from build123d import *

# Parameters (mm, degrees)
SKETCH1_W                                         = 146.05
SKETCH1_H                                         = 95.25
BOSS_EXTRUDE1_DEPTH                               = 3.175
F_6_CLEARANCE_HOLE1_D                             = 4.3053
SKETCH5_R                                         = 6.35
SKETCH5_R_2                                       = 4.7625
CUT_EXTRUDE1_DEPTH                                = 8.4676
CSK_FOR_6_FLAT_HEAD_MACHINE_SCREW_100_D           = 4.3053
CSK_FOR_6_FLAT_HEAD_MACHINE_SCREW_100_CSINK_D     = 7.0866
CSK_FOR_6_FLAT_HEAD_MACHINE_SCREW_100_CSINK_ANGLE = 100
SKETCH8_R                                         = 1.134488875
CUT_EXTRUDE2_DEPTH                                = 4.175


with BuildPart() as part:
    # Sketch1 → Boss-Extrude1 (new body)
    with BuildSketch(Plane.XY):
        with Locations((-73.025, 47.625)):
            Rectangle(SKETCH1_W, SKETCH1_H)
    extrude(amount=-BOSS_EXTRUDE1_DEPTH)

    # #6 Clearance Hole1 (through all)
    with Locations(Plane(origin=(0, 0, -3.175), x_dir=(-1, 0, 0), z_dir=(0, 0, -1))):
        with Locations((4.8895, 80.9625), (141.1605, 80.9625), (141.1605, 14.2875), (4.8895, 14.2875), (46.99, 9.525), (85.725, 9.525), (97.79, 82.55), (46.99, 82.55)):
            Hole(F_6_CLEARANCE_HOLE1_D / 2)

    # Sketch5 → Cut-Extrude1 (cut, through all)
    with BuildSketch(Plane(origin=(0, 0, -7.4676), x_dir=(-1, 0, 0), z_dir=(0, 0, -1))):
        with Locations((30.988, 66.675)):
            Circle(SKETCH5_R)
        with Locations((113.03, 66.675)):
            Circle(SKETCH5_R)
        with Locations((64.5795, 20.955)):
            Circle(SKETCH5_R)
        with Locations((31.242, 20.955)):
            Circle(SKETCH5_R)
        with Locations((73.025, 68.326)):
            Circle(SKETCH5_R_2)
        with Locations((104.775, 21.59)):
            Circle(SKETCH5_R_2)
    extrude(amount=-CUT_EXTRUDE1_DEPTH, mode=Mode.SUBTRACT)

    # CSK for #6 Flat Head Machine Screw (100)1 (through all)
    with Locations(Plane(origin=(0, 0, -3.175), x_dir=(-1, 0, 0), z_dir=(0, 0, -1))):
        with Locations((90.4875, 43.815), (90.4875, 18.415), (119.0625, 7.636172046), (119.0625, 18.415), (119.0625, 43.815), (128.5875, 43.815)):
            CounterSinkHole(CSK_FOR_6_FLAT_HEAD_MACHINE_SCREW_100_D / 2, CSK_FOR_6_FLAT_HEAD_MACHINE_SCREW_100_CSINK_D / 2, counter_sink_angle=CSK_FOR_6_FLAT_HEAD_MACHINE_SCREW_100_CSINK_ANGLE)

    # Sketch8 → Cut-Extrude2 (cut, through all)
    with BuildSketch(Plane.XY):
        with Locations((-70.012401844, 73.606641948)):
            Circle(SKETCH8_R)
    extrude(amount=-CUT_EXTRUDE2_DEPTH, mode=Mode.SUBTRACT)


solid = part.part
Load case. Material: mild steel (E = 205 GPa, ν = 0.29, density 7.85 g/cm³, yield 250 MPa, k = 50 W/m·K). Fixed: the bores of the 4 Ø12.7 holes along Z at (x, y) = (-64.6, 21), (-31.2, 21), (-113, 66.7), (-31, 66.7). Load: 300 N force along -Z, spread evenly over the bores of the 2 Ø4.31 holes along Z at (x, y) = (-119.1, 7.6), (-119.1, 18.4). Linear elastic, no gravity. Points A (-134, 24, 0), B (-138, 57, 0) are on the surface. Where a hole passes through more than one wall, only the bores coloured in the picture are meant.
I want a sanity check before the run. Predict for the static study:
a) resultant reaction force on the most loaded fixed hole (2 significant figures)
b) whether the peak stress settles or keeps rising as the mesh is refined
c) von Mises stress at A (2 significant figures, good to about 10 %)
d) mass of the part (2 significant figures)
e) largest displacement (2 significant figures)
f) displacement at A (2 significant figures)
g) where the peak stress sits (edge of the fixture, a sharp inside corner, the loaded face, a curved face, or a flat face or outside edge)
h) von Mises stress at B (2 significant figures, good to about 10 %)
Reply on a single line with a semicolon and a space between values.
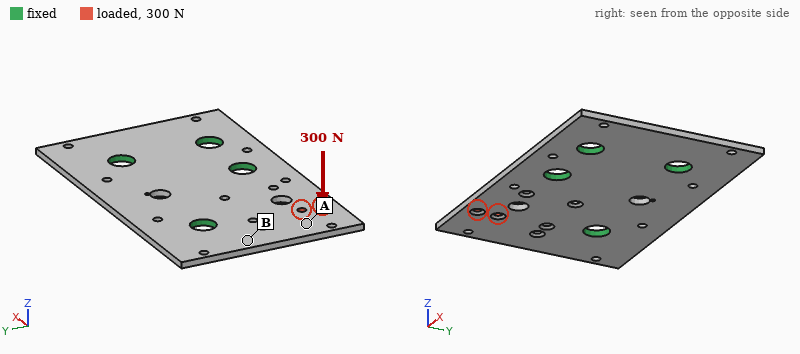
170 N; keeps rising; 17 MPa; 320 g; 0.33 mm; 0.17 mm; edge of the fixture; 47 MPa
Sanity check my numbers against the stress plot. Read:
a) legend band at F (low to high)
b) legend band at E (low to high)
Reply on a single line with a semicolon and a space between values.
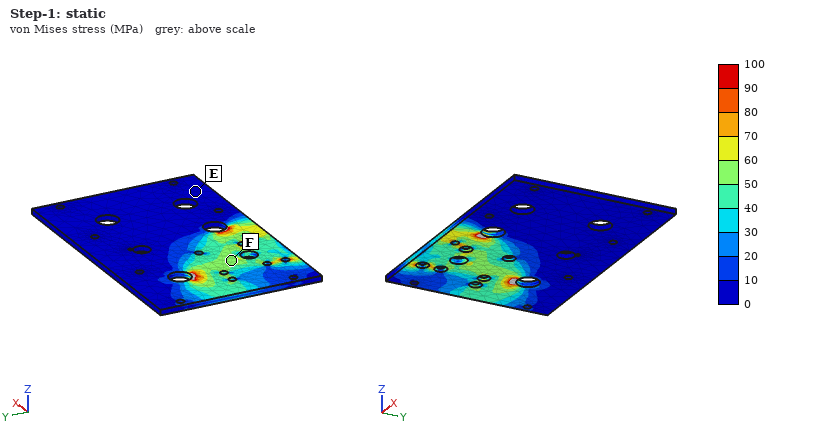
50 to 60 MPa; 0 to 10 MPa
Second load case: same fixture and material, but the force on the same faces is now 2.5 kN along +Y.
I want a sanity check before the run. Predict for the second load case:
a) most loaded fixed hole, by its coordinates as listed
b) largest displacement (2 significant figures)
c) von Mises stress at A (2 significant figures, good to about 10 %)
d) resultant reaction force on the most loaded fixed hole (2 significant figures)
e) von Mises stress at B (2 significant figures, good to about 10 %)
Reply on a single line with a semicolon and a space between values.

(-113, 66.7); 46 µm; 20 MPa; 2.2 kN; 13 MPa
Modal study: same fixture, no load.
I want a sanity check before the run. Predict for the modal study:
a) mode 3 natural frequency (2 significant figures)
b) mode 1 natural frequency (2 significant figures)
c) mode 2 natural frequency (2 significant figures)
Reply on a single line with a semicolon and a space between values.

2600 Hz; 970 Hz; 2500 Hz
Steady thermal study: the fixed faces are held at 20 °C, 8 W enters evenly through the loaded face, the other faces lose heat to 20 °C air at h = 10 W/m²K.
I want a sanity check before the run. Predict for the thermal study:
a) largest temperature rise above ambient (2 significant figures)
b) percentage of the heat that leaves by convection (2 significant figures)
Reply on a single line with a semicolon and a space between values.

41 K; 20 %
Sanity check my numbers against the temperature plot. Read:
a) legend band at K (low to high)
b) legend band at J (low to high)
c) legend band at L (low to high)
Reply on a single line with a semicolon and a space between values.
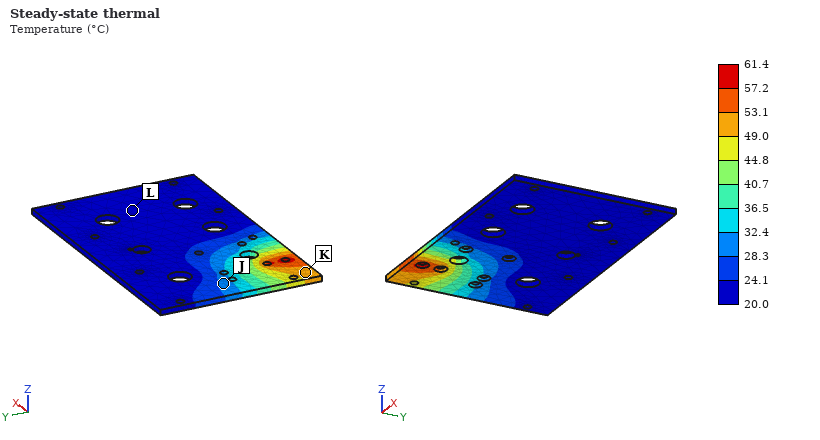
49.0 to 53.1 °C; 28.3 to 32.4 °C; 20.0 to 24.1 °C
